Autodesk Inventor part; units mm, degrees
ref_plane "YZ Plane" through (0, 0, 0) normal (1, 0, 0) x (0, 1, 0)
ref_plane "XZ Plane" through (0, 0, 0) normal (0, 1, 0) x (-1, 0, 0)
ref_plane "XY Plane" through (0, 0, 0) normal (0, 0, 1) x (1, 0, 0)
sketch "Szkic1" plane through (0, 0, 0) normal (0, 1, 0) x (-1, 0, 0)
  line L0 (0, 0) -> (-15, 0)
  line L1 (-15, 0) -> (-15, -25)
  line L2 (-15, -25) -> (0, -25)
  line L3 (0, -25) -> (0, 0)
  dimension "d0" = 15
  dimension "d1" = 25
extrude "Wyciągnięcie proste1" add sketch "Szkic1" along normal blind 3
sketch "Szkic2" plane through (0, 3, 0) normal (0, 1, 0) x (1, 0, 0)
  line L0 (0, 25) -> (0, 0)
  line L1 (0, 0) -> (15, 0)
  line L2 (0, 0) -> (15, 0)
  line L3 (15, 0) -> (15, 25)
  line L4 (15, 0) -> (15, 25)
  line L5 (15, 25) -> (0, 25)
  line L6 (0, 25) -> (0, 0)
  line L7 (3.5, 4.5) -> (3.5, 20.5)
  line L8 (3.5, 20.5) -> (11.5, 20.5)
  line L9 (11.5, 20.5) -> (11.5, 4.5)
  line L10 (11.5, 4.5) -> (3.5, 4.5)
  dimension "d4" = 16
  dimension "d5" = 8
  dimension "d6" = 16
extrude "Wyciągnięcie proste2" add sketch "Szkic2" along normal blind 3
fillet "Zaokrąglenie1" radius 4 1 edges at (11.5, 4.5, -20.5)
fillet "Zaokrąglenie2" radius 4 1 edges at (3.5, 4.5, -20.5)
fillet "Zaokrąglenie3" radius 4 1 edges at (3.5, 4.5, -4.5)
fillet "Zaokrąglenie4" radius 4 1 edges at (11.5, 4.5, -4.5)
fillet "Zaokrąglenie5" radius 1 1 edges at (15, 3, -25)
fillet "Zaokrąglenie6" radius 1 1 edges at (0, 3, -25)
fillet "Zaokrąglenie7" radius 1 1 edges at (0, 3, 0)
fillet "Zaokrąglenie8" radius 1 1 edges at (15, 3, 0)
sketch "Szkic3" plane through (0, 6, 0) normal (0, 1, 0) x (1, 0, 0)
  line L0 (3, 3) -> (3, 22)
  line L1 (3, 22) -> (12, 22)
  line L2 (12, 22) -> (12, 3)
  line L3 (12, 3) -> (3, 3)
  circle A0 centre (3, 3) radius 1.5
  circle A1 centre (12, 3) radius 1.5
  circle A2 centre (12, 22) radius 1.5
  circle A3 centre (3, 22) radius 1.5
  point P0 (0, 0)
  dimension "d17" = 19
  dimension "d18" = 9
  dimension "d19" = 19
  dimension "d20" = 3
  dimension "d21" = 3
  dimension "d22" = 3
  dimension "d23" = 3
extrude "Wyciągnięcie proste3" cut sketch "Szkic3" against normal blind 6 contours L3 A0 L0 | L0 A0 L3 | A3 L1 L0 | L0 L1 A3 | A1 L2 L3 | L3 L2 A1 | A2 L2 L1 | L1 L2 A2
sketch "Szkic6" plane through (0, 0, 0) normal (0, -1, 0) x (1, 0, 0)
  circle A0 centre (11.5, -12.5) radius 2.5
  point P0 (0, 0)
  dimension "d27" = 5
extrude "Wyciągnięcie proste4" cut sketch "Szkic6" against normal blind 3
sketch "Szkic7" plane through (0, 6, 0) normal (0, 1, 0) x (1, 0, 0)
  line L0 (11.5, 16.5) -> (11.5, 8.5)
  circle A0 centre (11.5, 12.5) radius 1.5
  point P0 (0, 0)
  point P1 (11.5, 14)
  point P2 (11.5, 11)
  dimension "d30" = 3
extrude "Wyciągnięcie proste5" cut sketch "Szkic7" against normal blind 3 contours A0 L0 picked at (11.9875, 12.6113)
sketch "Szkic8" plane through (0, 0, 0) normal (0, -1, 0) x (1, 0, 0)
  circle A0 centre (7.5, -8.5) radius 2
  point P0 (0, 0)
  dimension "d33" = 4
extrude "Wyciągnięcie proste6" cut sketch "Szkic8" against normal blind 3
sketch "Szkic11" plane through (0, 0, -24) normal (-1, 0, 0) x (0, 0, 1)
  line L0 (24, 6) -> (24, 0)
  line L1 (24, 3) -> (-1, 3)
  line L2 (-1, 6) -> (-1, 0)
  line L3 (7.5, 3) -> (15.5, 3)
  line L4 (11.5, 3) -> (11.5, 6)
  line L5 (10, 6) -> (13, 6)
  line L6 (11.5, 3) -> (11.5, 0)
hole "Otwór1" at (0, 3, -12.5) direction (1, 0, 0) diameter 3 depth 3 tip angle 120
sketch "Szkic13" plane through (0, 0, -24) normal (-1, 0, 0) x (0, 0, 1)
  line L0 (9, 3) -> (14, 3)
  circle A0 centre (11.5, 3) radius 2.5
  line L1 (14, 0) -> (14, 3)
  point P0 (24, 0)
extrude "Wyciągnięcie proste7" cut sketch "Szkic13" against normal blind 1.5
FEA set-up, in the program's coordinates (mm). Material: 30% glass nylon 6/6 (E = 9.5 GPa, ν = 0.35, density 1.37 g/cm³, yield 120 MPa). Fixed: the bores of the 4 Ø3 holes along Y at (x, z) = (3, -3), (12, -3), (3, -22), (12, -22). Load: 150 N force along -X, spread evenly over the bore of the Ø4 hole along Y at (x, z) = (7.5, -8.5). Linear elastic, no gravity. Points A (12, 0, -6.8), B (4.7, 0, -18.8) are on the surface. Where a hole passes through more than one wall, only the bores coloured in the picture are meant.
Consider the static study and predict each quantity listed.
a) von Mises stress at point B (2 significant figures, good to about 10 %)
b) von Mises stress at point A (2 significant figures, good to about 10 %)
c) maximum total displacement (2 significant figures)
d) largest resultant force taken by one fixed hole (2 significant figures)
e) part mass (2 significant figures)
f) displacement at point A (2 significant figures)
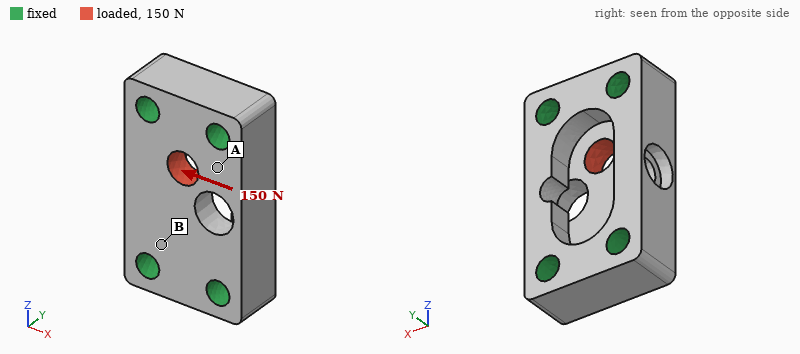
1.3 MPa
3.8 MPa
6.0 µm
64 N
2.2 g
2.2 µm
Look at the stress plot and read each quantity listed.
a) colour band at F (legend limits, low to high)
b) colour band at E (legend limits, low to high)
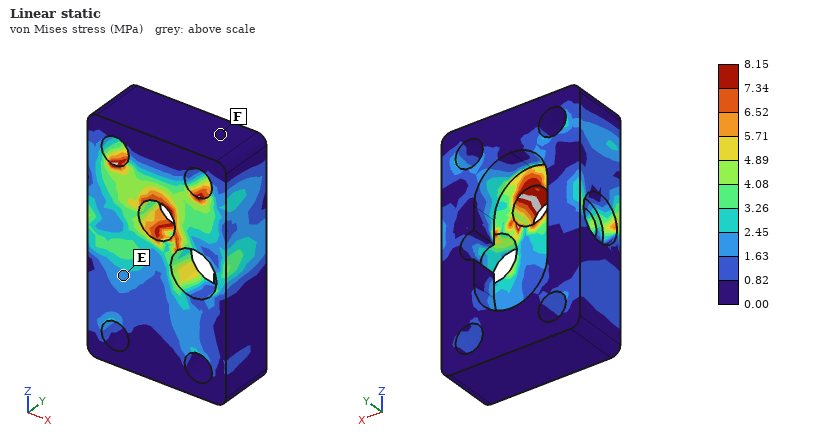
0.00 to 0.82 MPa
1.63 to 2.45 MPa
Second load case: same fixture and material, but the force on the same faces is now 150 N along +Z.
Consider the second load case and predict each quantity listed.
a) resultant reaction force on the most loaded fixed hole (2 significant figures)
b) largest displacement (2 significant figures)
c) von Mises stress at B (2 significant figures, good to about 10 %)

59 N
3.6 µm
1.4 MPa
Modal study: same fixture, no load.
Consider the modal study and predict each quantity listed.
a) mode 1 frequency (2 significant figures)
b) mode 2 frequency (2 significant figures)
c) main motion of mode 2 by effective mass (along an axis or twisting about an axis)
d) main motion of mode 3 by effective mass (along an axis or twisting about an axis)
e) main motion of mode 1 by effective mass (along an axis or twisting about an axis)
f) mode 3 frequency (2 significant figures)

34 kHz
37 kHz
along X
along X
along Y
41 kHz
